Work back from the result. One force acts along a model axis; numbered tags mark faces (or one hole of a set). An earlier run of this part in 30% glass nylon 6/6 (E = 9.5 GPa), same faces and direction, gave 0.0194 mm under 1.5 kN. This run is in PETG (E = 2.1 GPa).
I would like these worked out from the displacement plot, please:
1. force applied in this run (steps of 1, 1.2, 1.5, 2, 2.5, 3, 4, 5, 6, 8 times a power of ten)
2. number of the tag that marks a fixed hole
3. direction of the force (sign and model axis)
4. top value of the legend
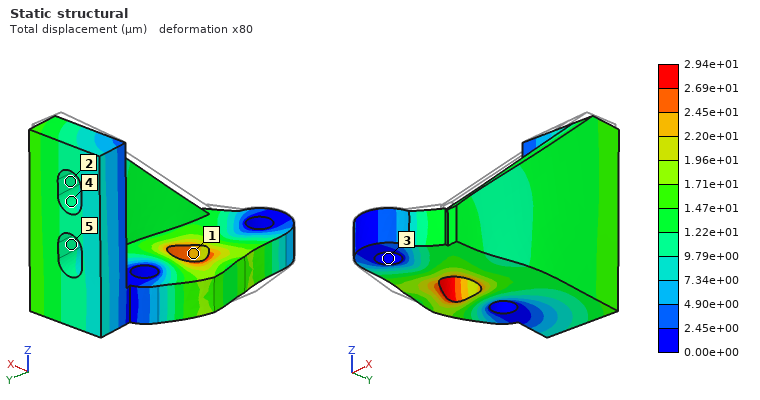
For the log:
500 N
3
+Y
2.94e+01 µm
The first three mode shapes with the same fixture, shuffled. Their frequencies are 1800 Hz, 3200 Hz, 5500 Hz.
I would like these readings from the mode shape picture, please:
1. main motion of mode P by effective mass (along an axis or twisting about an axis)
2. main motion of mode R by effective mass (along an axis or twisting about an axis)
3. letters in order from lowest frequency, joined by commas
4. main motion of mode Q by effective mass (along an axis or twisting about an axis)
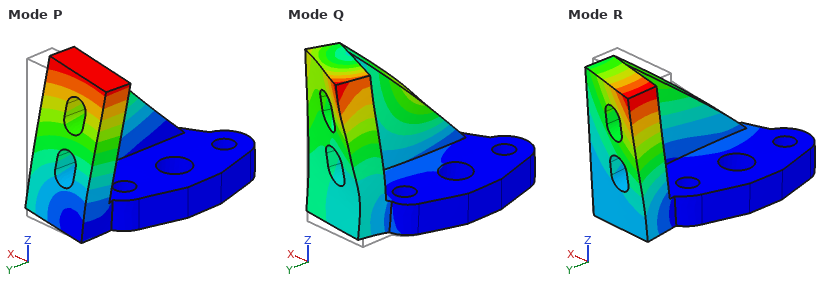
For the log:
along X
along Y
P, R, Q
along Z
